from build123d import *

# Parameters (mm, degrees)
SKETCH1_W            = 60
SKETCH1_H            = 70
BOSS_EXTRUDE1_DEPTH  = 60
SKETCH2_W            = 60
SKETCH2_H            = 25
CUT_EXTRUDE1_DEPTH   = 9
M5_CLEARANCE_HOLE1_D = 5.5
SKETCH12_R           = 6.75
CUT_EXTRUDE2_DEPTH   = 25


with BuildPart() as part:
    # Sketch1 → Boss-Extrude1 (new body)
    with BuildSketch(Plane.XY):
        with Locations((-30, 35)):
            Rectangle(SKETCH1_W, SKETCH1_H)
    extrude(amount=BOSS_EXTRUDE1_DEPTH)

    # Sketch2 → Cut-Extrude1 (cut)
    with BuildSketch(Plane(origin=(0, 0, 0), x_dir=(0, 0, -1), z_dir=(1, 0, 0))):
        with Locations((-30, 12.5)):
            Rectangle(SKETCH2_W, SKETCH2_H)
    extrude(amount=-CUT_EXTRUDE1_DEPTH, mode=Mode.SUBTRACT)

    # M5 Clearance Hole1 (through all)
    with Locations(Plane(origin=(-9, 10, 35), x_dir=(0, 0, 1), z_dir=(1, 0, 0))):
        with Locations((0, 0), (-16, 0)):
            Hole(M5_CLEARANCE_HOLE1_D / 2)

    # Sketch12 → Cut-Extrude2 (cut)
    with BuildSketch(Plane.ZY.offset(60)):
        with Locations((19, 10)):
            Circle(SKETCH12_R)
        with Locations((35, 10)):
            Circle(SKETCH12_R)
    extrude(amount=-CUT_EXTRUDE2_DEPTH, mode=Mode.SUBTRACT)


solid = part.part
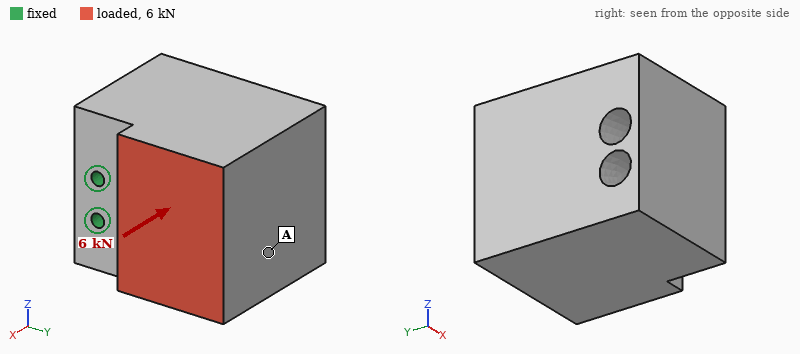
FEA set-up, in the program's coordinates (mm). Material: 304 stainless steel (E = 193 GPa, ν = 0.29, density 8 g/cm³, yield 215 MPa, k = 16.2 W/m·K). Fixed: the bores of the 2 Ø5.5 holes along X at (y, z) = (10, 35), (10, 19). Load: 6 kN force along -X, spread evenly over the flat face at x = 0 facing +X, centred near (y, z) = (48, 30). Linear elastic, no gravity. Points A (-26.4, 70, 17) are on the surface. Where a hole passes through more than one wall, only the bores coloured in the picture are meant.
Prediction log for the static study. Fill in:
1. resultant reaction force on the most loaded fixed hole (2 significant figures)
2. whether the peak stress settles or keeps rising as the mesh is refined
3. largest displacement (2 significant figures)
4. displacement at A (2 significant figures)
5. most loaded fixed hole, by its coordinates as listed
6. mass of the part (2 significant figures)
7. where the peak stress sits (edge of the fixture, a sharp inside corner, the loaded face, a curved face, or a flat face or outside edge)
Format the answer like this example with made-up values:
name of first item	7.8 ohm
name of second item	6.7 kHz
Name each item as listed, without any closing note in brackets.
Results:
resultant reaction force on the most loaded fixed hole	3.4 kN
whether the peak stress settles or keeps rising as the mesh is refined	keeps rising
largest displacement	17 µm
displacement at A	14 µm
most loaded fixed hole, by its coordinates as listed	(10, 35)
mass of the part	1.8 kg
where the peak stress sits	edge of the fixture
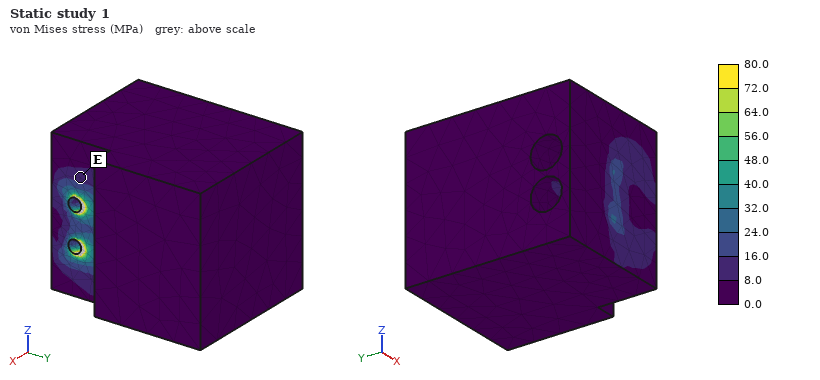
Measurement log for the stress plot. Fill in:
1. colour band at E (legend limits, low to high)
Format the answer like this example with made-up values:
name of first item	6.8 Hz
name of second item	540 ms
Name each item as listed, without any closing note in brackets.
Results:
colour band at E	8.0 to 16.0 MPa
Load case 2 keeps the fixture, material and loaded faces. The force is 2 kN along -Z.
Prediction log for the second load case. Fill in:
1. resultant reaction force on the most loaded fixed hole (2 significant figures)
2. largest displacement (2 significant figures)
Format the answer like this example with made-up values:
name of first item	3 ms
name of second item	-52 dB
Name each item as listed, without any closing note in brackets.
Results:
resultant reaction force on the most loaded fixed hole	3.8 kN
largest displacement	6.0 µm
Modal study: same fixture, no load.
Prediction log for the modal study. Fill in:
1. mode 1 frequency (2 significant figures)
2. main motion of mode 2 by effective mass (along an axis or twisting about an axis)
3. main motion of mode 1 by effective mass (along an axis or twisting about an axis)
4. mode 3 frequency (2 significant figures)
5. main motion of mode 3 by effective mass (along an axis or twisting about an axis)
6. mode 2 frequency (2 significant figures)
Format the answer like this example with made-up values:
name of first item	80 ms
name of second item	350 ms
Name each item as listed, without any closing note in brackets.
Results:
mode 1 frequency	3000 Hz
main motion of mode 2 by effective mass	along Z
main motion of mode 1 by effective mass	along X
mode 3 frequency	5800 Hz
main motion of mode 3 by effective mass	twisting about Y
mode 2 frequency	3300 Hz
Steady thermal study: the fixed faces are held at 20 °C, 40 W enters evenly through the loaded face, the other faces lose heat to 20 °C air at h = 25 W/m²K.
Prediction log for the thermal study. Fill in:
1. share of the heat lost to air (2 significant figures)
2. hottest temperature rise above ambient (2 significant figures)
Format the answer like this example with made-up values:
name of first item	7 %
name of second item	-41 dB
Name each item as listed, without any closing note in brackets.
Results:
share of the heat lost to air	28 %
hottest temperature rise above ambient	49 K
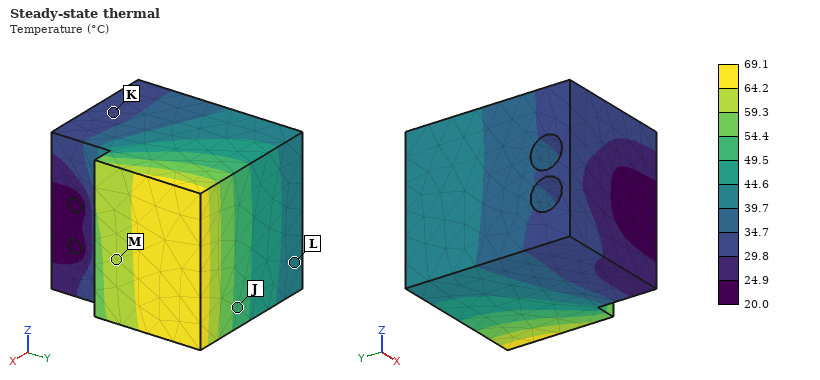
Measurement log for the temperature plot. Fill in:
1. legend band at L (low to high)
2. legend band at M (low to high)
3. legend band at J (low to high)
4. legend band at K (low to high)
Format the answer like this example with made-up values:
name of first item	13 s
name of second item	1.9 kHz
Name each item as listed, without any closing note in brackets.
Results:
legend band at L	39.7 to 44.6 °C
legend band at M	59.3 to 64.2 °C
legend band at J	49.5 to 54.4 °C
legend band at K	29.8 to 34.7 °C
